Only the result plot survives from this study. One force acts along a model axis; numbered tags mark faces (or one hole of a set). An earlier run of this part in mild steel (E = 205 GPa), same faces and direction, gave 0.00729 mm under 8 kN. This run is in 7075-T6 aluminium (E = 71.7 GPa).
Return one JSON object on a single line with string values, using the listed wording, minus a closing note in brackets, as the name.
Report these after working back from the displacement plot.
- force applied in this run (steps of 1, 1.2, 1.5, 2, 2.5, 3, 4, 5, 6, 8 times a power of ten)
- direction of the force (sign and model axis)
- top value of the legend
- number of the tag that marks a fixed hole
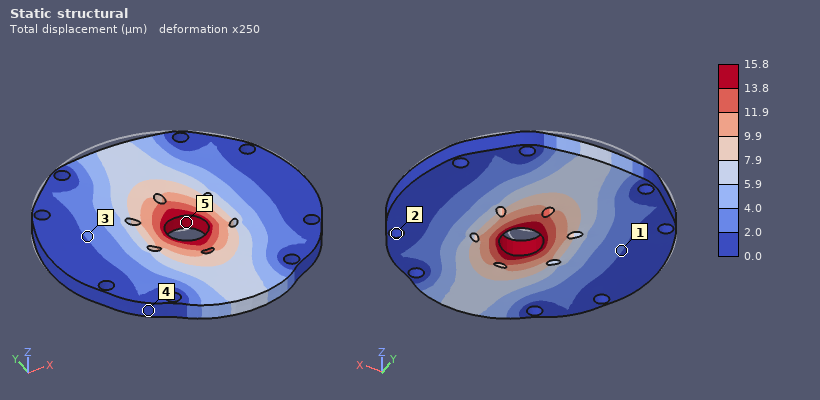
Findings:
{"force applied in this run": "6 kN", "direction of the force": "-Y", "top value of the legend": "15.8 µm", "number of the tag that marks a fixed hole": "2"}
